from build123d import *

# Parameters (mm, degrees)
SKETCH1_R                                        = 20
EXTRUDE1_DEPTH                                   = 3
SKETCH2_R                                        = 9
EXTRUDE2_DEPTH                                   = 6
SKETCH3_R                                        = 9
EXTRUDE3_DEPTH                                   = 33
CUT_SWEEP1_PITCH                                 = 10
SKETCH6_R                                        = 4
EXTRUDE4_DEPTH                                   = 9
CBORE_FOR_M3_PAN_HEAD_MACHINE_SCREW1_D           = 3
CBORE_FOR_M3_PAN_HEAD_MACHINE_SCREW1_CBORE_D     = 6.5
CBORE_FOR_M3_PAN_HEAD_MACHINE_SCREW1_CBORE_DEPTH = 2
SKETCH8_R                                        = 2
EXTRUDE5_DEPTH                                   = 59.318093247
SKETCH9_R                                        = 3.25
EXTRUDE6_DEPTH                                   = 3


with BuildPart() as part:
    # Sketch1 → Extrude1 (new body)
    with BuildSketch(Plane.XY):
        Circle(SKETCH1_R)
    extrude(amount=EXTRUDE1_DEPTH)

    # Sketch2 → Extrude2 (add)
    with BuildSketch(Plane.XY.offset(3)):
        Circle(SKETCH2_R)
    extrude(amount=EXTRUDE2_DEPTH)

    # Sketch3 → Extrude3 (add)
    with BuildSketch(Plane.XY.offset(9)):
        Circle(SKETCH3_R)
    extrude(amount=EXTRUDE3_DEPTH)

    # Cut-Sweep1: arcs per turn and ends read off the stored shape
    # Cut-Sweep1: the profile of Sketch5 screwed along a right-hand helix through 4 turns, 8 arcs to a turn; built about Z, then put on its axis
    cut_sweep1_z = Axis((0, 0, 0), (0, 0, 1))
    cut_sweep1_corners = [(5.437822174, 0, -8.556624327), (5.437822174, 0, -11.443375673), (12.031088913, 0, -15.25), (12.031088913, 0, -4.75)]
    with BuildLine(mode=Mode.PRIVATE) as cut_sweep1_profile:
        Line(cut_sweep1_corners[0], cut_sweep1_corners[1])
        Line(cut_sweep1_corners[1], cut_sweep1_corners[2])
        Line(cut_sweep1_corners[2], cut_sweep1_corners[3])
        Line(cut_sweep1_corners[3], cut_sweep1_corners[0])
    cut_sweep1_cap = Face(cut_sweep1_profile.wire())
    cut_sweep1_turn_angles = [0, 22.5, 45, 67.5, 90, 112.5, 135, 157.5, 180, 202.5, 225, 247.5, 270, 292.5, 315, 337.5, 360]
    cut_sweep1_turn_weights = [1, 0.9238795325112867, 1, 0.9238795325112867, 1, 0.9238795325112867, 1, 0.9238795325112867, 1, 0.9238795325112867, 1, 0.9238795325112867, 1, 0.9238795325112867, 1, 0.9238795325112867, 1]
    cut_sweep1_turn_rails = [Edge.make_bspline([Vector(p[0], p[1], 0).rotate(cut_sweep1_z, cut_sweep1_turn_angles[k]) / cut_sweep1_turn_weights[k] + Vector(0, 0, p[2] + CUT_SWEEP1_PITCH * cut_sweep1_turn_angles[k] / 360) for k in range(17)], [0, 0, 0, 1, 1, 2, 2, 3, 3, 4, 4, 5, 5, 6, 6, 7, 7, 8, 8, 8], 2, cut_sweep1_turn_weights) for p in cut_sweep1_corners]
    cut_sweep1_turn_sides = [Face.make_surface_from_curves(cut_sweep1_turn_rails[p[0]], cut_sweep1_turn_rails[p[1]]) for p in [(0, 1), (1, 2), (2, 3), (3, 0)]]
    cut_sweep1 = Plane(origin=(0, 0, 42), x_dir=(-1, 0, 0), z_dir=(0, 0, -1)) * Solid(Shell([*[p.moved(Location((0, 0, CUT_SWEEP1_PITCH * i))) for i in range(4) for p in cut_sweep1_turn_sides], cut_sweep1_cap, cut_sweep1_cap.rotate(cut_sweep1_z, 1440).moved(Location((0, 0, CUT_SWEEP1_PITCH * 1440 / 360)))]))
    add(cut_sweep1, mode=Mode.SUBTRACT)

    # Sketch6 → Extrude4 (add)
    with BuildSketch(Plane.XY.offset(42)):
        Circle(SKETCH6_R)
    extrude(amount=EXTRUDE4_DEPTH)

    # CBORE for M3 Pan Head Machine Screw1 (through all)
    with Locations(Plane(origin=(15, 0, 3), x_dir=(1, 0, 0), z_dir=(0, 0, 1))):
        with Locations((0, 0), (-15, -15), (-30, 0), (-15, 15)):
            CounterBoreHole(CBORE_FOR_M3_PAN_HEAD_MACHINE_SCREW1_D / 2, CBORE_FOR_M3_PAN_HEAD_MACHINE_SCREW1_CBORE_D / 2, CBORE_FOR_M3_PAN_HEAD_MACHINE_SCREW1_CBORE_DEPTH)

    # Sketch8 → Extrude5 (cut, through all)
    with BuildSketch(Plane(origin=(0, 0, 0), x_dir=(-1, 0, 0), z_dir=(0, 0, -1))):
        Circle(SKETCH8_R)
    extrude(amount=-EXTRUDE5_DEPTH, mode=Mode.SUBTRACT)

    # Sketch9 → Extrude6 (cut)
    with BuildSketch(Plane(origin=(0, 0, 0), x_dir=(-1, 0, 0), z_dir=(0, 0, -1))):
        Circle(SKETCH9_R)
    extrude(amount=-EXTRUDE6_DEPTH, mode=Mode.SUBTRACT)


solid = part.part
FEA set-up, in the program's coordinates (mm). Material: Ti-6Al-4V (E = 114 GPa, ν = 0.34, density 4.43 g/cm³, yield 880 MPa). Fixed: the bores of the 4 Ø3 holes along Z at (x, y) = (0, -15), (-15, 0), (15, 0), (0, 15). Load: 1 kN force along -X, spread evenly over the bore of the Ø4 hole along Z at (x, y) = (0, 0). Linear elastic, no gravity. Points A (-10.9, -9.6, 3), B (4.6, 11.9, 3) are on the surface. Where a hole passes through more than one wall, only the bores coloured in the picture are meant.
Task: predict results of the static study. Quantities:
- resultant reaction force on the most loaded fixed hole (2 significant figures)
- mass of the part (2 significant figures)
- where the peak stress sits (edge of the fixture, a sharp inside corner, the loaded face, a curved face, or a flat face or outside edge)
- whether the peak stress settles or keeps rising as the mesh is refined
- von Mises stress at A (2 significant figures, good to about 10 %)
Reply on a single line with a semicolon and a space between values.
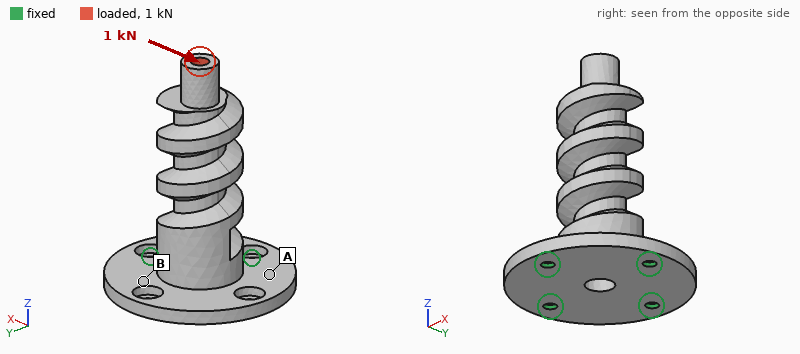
1.1 kN; 47 g; edge of the fixture; keeps rising; 47 MPa
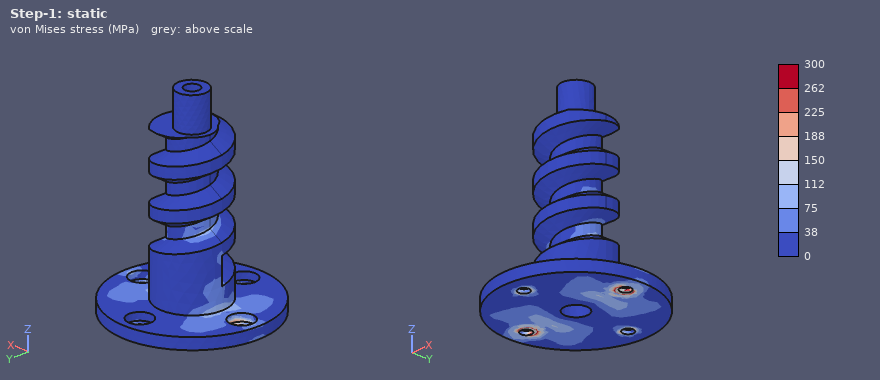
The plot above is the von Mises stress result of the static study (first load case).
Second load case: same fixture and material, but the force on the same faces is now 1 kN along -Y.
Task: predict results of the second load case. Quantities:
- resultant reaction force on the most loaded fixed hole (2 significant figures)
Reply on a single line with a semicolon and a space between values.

1.2 kN
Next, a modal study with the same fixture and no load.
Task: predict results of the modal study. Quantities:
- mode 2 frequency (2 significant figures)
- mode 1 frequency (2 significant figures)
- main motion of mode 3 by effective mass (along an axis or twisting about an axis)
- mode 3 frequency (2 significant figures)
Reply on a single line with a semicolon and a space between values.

3300 Hz; 3200 Hz; along Z; 9200 Hz
